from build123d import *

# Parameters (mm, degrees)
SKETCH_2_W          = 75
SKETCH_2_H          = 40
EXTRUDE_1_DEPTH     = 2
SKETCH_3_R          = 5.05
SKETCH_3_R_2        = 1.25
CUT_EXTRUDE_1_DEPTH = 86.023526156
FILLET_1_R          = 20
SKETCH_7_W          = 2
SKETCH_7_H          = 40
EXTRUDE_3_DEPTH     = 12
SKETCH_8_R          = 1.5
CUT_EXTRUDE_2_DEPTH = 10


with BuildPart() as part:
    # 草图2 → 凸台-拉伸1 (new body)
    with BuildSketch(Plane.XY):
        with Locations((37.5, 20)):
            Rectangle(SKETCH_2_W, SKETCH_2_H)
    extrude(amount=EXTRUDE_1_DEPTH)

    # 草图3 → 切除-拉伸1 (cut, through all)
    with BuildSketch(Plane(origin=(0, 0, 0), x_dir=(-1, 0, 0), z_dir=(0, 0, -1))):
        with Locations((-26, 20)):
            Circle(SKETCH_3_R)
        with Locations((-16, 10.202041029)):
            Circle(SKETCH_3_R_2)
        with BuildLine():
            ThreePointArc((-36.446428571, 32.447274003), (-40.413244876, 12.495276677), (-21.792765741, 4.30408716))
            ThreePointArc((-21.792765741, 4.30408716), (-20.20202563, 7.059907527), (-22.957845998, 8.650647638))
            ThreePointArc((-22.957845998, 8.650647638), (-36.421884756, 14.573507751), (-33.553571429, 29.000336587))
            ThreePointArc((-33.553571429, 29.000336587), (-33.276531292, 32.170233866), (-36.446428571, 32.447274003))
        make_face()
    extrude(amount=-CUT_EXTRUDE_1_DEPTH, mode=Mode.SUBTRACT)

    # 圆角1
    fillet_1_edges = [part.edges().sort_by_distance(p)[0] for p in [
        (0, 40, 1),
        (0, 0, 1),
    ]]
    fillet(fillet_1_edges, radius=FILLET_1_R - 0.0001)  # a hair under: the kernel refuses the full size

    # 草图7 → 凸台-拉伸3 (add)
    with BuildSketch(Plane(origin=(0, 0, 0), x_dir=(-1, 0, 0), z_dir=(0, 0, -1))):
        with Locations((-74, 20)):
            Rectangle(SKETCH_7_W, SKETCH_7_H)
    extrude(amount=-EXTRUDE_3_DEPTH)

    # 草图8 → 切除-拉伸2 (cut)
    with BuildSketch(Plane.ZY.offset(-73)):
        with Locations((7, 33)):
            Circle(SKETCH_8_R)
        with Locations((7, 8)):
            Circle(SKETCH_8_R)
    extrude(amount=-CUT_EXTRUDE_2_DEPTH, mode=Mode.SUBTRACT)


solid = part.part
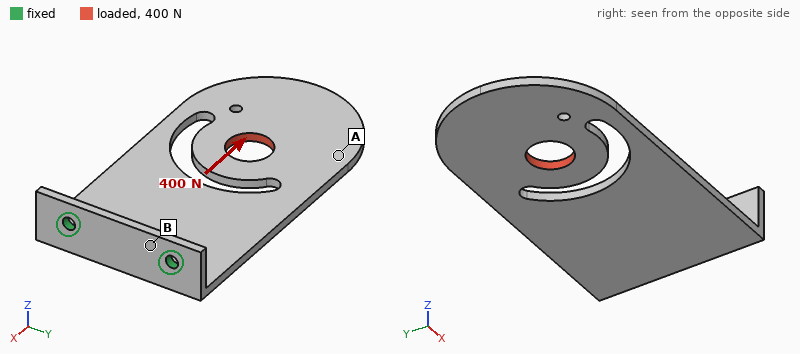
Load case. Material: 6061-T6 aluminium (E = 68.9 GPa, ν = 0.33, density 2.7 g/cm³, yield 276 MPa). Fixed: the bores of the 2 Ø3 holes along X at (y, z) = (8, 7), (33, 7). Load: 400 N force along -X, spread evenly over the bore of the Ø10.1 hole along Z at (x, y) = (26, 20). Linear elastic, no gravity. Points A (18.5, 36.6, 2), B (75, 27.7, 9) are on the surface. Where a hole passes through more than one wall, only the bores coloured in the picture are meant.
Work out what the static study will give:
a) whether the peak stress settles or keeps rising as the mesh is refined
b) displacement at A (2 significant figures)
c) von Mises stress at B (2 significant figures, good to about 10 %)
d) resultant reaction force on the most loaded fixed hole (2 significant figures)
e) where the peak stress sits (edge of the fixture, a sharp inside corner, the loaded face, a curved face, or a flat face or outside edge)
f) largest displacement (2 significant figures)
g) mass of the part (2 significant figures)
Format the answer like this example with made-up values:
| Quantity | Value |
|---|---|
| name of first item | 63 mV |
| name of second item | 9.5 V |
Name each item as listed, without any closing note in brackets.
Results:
| Quantity | Value |
|---|---|
| whether the peak stress settles or keeps rising as the mesh is refined | keeps rising |
| displacement at A | 0.24 mm |
| von Mises stress at B | 20 MPa |
| resultant reaction force on the most loaded fixed hole | 210 N |
| where the peak stress sits | edge of the fixture |
| largest displacement | 0.32 mm |
| mass of the part | 16 g |
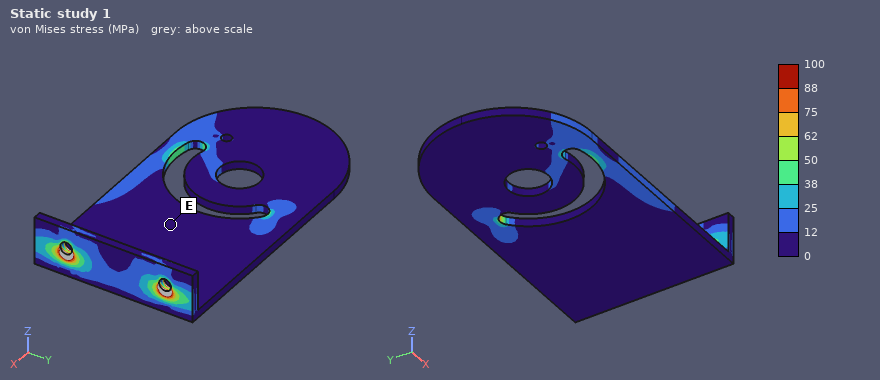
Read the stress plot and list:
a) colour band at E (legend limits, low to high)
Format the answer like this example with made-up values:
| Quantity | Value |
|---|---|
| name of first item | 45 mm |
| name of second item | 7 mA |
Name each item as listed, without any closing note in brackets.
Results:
| Quantity | Value |
|---|---|
| colour band at E | 0 to 12 MPa |
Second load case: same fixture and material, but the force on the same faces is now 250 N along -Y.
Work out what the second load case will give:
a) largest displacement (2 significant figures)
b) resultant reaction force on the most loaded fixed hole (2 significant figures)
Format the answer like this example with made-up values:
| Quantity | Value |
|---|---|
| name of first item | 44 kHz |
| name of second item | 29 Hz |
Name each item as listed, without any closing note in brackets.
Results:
| Quantity | Value |
|---|---|
| largest displacement | 0.25 mm |
| resultant reaction force on the most loaded fixed hole | 470 N |
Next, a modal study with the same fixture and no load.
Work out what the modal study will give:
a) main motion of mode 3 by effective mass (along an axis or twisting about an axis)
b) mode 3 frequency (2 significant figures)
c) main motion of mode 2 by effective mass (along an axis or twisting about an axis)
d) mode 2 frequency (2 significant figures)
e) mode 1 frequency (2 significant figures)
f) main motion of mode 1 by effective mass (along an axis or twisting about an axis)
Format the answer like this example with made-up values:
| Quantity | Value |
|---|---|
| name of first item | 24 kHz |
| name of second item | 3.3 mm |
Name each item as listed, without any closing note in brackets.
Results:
| Quantity | Value |
|---|---|
| main motion of mode 3 by effective mass | along Z |
| mode 3 frequency | 1400 Hz |
| main motion of mode 2 by effective mass | twisting about X |
| mode 2 frequency | 1200 Hz |
| mode 1 frequency | 290 Hz |
| main motion of mode 1 by effective mass | along Z |
